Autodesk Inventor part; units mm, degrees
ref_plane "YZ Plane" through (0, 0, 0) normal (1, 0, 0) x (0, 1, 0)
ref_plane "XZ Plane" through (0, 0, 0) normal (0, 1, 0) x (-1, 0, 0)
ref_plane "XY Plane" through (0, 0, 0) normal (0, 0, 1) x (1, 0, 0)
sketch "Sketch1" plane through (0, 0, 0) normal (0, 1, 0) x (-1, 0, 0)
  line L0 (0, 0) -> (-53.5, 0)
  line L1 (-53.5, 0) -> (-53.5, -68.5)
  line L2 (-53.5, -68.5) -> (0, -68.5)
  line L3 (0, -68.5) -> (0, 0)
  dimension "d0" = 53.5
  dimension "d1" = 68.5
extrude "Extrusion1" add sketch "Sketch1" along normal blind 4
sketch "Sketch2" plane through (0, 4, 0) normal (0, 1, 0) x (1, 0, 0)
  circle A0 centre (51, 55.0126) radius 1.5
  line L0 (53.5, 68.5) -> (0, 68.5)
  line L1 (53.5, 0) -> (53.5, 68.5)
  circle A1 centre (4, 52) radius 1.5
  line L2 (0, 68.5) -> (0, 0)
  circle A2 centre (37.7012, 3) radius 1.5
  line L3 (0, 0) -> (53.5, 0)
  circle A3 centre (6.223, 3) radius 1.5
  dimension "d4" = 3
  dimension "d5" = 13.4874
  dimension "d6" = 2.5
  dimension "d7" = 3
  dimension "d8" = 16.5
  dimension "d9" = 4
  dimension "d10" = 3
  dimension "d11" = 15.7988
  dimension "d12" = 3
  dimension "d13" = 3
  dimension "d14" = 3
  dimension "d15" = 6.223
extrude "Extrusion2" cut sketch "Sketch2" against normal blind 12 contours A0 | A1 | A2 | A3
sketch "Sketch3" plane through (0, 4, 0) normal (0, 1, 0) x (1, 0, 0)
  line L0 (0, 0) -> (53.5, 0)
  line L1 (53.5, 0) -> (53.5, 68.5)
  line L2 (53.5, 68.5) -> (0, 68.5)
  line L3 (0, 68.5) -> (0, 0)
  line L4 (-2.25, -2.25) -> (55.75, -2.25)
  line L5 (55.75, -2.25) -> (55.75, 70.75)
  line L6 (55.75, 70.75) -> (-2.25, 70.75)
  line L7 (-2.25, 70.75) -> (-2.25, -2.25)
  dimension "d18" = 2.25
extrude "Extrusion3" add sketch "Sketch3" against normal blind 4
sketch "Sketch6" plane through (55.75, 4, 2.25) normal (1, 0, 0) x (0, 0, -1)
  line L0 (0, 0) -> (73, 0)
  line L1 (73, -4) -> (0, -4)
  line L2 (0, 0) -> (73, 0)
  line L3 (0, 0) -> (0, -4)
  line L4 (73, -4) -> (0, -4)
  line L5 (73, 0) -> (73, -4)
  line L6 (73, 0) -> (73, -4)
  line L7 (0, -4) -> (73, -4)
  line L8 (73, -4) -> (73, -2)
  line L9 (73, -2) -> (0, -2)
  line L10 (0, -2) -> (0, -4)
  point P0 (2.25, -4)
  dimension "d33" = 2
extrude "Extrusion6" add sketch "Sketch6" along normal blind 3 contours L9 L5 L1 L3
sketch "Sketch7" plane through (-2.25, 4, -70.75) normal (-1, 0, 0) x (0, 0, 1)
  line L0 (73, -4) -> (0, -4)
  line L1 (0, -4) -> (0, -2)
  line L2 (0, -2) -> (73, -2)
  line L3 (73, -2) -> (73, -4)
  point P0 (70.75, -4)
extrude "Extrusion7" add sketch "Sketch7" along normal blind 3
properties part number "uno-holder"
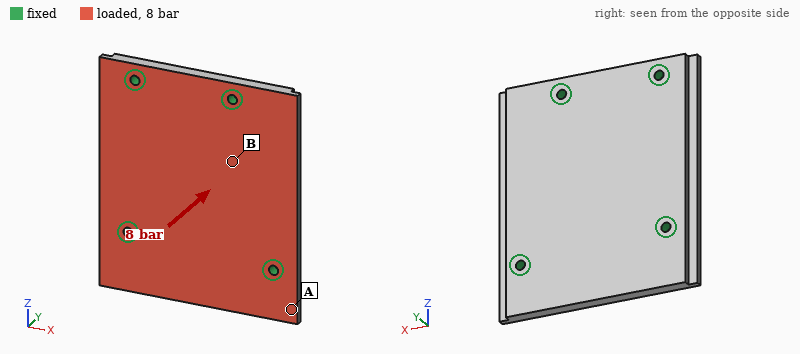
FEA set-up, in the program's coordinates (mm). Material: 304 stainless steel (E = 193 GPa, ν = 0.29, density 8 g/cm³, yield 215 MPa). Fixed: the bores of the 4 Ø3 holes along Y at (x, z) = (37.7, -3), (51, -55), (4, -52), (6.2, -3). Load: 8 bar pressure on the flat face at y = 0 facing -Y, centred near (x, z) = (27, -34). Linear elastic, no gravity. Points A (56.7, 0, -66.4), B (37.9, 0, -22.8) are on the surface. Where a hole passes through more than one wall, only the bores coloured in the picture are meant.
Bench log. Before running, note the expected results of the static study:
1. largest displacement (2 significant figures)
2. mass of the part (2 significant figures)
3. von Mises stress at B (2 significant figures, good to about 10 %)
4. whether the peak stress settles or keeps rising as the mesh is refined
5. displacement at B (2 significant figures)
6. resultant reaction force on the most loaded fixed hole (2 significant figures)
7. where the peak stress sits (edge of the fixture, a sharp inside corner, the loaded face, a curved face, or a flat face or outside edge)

35 µm
140 g
37 MPa
keeps rising
23 µm
1.1 kN
edge of the fixture
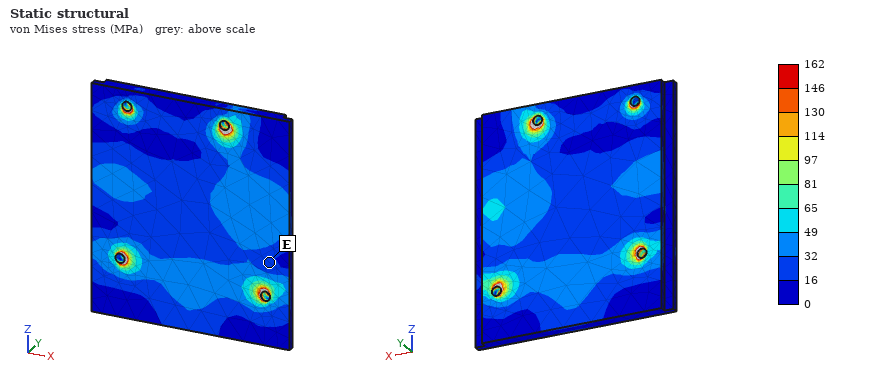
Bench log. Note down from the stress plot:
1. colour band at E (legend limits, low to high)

16 to 32 MPa
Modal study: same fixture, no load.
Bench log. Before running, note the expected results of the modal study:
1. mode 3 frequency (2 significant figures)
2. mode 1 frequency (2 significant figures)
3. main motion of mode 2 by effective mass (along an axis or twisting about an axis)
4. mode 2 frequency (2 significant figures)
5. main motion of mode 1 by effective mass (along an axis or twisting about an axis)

6700 Hz
5500 Hz
along Y
6200 Hz
along Y
